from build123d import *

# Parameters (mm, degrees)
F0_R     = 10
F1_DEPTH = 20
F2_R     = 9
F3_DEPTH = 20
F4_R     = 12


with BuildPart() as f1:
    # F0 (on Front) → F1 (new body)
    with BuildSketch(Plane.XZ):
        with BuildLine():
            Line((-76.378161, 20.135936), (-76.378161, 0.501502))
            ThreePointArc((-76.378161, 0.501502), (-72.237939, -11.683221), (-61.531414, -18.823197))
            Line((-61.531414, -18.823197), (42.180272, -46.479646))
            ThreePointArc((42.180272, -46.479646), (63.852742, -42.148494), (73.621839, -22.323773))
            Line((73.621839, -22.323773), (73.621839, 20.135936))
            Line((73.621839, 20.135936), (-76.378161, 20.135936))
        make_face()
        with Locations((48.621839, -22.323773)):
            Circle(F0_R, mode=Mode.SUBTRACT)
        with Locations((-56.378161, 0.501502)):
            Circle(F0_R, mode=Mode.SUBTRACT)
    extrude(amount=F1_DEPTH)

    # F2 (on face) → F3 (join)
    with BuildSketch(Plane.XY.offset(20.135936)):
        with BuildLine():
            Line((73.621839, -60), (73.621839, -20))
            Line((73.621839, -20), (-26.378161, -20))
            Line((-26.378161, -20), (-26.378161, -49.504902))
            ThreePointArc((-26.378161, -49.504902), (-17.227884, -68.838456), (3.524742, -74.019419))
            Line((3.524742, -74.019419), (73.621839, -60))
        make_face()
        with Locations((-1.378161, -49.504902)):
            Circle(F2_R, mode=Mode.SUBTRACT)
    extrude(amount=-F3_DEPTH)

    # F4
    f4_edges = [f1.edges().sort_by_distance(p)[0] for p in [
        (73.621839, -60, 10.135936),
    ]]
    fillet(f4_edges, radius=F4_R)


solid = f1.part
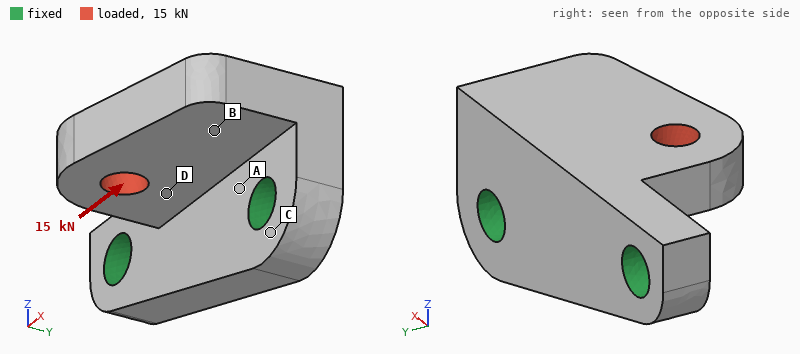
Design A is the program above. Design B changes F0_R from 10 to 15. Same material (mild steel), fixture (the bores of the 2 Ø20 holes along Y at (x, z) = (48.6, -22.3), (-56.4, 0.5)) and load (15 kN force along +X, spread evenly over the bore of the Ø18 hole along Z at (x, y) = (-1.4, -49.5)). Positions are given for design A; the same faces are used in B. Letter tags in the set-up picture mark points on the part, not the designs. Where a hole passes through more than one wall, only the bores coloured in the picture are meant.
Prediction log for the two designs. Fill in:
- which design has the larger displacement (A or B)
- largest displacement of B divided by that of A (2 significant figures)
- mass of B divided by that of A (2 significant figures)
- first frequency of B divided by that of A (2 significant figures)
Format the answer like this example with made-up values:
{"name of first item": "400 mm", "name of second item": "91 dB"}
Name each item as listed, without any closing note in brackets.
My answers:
{"which design has the larger displacement": "A", "largest displacement of B divided by that of A": "0.78", "mass of B divided by that of A": "0.93", "first frequency of B divided by that of A": "1.1"}
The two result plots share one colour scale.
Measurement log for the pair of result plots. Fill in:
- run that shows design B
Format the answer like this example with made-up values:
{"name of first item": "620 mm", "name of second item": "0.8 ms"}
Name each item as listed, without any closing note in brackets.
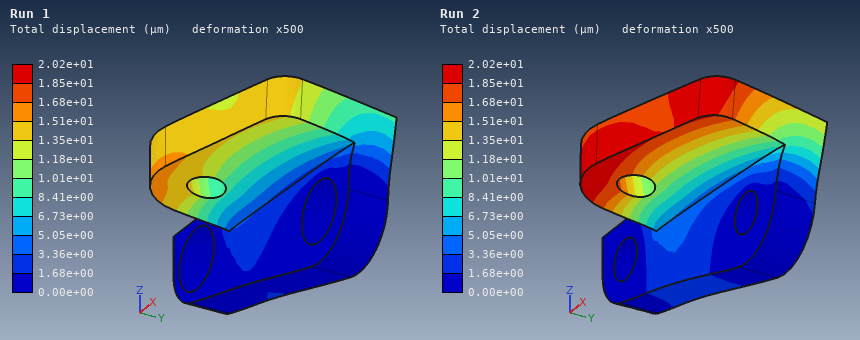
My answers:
{"run that shows design B": "Run 1"}
